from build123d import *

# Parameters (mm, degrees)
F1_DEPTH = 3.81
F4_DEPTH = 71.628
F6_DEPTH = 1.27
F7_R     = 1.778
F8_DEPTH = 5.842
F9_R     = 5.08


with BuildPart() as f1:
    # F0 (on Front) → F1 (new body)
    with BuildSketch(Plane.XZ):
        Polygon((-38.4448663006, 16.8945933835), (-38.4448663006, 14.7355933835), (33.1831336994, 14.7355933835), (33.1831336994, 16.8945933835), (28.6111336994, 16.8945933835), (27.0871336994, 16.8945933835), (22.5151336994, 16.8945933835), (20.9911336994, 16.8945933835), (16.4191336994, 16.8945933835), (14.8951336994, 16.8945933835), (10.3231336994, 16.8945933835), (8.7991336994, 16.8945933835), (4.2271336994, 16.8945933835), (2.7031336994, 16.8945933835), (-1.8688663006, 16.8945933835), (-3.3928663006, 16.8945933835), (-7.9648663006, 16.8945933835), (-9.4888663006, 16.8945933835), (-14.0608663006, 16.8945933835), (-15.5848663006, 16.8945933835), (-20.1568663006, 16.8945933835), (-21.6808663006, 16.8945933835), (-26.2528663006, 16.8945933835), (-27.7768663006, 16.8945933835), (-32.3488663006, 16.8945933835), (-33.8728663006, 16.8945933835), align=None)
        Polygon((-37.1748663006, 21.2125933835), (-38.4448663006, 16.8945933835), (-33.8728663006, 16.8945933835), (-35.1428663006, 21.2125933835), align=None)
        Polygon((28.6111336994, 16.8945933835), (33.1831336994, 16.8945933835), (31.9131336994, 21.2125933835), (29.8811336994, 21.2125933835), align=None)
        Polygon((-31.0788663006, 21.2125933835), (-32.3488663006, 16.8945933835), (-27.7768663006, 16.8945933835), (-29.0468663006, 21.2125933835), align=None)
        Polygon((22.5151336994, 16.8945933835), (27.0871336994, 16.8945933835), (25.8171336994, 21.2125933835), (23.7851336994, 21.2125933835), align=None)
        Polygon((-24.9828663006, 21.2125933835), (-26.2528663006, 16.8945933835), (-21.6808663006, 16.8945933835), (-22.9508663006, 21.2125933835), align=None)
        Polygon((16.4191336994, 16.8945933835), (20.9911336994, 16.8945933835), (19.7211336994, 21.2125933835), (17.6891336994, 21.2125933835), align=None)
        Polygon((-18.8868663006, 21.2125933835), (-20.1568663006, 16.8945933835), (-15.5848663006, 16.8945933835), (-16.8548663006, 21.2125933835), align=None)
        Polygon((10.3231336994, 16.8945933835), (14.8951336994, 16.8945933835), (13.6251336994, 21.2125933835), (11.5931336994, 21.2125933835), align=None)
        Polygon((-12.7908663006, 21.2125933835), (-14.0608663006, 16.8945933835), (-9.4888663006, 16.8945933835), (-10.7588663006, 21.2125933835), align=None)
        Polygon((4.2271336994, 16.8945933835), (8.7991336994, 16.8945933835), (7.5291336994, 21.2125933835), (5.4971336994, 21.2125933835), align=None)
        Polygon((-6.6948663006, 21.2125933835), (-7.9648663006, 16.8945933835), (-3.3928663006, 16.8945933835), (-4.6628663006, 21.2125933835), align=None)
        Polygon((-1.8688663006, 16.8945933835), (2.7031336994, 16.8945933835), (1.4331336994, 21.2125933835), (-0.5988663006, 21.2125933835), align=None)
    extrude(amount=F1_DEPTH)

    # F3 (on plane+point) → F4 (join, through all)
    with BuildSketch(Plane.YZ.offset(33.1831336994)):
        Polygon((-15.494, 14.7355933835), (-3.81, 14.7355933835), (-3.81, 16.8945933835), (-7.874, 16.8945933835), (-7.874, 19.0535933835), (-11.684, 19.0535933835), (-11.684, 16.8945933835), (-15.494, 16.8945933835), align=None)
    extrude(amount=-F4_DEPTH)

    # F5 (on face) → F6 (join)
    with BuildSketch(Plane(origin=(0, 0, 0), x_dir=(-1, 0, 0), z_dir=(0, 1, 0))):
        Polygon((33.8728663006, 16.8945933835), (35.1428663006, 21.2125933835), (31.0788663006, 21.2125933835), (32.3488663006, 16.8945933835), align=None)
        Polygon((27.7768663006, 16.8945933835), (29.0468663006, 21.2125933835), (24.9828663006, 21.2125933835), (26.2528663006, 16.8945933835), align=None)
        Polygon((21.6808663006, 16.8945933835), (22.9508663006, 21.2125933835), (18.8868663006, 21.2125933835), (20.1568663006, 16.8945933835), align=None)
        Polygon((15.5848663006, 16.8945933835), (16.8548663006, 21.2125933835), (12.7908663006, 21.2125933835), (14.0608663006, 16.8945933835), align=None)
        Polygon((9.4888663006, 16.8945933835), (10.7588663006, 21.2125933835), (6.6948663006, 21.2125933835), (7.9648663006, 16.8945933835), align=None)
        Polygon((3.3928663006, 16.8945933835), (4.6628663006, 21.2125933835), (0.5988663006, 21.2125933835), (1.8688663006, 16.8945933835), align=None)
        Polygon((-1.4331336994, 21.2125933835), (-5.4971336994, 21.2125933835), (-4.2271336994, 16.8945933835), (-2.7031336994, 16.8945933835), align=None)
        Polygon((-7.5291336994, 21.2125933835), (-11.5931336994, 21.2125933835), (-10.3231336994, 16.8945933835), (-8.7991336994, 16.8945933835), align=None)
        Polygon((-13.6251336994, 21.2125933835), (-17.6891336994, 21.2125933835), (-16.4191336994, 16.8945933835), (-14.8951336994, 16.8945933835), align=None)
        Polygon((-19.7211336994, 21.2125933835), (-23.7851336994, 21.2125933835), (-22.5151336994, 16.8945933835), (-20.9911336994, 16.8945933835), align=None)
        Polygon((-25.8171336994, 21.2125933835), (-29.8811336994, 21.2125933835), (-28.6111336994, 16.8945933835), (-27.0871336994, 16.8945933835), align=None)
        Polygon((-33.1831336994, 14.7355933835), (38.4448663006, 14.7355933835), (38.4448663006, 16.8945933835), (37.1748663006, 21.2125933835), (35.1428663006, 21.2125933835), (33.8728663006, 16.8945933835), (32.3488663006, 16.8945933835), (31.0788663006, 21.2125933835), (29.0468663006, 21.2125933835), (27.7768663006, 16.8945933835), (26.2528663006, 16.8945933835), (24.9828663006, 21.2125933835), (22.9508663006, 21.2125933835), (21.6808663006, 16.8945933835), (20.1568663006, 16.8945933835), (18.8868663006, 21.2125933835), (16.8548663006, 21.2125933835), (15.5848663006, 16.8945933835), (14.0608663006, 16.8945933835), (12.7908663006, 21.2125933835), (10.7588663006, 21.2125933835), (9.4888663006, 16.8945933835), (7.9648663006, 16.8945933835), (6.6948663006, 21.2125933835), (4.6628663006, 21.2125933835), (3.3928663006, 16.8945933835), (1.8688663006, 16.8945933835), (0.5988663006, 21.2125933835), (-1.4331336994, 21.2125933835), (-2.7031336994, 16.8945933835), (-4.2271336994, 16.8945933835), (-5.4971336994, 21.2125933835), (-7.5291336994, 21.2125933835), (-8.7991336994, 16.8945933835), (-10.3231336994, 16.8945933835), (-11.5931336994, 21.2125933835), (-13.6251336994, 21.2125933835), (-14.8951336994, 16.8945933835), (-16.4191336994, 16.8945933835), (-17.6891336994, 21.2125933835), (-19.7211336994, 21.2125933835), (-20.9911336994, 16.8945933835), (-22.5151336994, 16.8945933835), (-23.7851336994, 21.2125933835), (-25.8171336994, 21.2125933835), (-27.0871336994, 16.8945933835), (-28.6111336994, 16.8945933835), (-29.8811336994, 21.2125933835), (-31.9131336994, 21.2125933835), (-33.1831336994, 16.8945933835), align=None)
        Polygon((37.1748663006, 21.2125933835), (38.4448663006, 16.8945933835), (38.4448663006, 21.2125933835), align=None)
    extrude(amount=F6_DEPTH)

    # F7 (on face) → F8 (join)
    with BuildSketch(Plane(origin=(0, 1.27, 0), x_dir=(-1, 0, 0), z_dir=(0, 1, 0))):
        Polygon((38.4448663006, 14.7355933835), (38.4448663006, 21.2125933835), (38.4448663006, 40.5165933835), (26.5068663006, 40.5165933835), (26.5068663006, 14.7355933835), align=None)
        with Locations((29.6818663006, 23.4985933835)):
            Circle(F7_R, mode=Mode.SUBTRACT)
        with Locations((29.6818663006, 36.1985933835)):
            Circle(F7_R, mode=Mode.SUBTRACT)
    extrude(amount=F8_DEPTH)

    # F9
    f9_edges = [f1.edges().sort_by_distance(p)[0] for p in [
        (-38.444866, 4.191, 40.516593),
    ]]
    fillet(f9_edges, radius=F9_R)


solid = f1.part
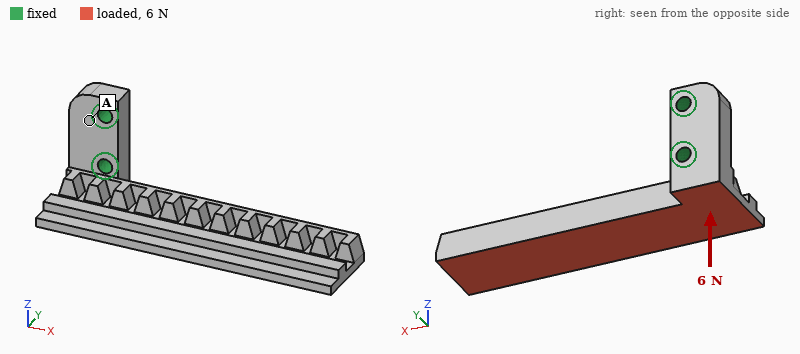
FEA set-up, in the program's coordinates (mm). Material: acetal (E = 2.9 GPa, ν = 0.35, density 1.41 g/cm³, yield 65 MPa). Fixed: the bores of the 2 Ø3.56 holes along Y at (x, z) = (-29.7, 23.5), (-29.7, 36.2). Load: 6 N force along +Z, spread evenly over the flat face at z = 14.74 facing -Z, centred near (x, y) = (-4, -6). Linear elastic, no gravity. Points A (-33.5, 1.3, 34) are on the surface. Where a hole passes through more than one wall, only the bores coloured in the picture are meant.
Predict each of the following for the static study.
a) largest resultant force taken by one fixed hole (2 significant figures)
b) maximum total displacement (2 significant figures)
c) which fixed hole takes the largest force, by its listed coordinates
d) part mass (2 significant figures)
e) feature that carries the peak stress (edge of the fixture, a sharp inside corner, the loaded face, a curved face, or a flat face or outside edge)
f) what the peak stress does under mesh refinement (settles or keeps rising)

15 N
0.75 mm
(-29.7, 23.5)
8.3 g
a sharp inside corner
keeps rising
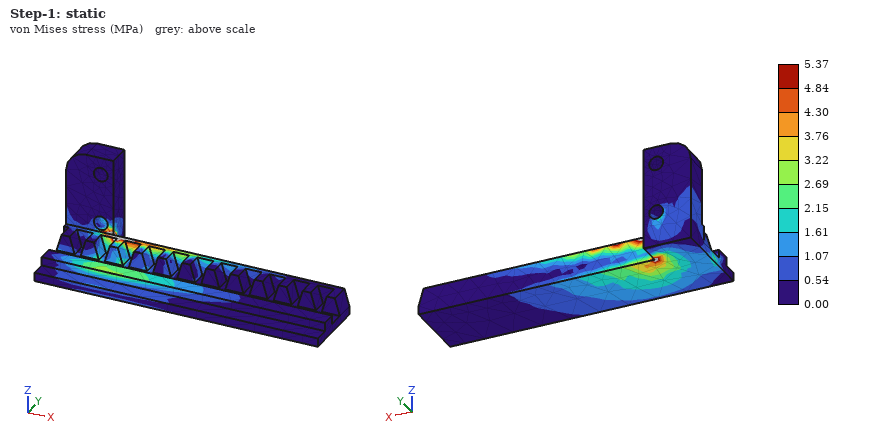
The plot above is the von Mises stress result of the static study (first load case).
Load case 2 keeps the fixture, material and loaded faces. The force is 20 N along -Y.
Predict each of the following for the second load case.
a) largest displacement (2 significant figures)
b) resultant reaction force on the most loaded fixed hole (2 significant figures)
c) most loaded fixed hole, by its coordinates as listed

0.77 mm
21 N
(-29.7, 23.5)
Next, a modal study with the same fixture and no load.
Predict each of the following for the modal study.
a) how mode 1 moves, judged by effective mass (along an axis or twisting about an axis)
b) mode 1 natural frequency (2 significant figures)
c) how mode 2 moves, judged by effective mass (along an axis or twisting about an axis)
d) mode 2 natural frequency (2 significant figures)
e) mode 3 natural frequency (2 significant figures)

along Z
230 Hz
along Y
430 Hz
930 Hz
